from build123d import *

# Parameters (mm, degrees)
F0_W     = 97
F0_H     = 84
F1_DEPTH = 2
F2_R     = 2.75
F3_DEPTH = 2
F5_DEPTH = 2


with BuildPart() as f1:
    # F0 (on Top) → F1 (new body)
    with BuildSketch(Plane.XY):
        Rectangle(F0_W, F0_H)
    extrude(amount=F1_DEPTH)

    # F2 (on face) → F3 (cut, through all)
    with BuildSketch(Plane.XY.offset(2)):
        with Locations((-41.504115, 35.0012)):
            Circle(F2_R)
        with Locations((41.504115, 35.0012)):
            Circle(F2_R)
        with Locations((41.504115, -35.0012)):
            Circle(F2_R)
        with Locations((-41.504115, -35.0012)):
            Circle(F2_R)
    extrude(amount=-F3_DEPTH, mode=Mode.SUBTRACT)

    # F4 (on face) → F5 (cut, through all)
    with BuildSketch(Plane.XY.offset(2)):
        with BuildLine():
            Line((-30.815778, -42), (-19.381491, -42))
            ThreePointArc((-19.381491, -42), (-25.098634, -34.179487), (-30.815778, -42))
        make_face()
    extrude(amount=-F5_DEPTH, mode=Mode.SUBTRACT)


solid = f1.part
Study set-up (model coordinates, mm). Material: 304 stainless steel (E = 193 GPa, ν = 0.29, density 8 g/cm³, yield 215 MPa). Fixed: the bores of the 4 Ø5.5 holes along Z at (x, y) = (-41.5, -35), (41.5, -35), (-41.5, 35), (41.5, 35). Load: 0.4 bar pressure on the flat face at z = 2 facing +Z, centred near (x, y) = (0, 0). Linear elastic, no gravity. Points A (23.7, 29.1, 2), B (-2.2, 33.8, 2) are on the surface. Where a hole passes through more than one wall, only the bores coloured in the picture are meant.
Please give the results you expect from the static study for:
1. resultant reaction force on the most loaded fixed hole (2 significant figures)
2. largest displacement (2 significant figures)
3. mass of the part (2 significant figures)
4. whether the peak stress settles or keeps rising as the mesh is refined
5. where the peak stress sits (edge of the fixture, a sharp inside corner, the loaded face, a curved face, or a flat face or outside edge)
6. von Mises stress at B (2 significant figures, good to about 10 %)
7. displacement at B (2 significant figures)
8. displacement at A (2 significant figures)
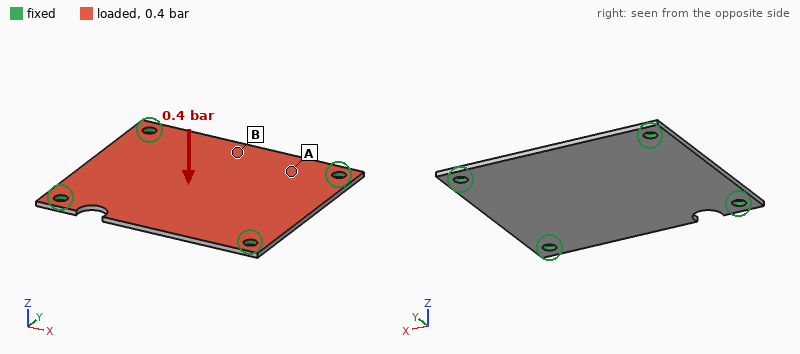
81 N
69 µm
130 g
keeps rising
edge of the fixture
20 MPa
48 µm
27 µm
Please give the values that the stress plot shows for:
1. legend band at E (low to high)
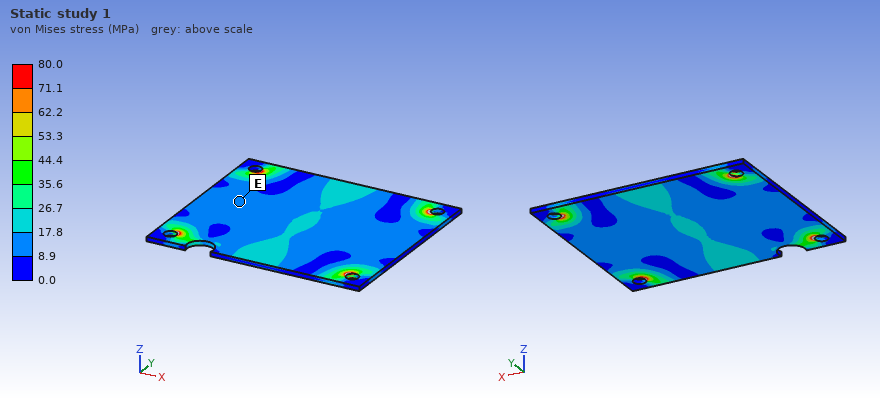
8.9 to 17.8 MPa
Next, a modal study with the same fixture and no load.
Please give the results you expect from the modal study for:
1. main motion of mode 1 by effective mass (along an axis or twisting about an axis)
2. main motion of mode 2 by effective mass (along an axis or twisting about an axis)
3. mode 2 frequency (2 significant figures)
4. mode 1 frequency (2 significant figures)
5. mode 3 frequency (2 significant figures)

along Z
twisting about X
1800 Hz
1200 Hz
2200 Hz
